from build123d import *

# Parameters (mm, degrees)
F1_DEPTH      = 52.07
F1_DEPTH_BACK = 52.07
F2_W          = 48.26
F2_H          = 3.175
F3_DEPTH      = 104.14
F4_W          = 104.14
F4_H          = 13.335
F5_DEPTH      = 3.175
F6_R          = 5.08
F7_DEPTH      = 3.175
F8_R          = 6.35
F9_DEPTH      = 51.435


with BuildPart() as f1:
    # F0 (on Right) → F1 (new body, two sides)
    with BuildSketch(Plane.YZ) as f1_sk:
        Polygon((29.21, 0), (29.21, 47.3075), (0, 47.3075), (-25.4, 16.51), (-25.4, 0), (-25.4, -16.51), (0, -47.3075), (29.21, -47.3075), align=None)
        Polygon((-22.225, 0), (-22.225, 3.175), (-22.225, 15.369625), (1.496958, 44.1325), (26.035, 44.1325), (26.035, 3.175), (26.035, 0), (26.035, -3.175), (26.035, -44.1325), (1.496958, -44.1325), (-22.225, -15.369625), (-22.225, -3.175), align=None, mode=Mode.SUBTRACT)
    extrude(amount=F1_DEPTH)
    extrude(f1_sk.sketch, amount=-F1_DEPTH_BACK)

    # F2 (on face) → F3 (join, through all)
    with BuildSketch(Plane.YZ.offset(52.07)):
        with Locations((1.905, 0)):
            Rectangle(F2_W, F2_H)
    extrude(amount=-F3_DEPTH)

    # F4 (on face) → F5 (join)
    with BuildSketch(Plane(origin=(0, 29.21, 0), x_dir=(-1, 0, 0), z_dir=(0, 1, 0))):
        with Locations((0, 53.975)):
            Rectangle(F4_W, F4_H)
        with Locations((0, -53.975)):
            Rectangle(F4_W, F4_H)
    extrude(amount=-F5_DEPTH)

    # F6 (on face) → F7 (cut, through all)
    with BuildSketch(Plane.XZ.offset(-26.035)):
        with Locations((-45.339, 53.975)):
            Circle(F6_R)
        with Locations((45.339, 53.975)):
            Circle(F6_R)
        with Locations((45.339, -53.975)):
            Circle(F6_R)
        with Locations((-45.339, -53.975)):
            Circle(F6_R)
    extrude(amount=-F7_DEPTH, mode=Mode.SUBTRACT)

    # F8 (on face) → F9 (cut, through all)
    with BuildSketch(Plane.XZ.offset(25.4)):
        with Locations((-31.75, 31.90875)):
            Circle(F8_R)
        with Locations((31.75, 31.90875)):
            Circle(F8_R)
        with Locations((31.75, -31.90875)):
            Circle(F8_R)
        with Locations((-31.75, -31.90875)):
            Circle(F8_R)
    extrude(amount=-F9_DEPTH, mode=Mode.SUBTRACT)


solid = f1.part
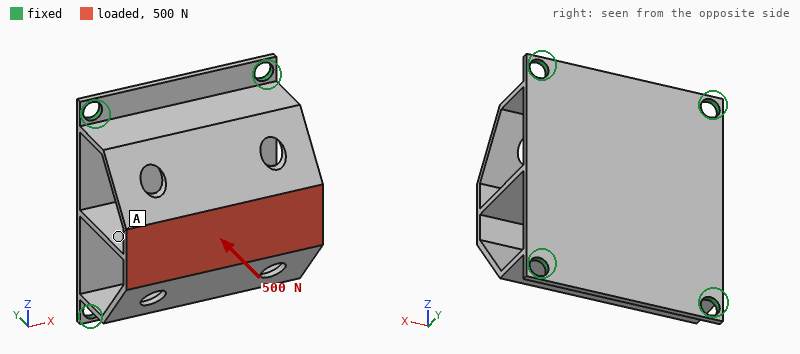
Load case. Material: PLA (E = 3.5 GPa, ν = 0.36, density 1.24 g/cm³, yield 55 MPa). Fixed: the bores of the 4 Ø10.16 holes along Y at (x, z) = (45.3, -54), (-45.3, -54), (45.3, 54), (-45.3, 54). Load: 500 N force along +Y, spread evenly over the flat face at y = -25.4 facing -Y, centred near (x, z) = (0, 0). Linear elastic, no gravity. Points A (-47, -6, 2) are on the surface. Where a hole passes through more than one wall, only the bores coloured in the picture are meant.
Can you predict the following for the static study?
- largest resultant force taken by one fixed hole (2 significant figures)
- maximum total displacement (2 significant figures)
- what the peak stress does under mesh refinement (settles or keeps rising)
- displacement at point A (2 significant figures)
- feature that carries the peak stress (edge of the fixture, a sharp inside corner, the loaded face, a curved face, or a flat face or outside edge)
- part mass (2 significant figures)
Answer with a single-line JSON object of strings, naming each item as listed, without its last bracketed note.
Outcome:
{"largest resultant force taken by one fixed hole": "140 N", "maximum total displacement": "0.51 mm", "what the peak stress does under mesh refinement": "keeps rising", "displacement at point A": "0.50 mm", "feature that carries the peak stress": "edge of the fixture", "part mass": "130 g"}
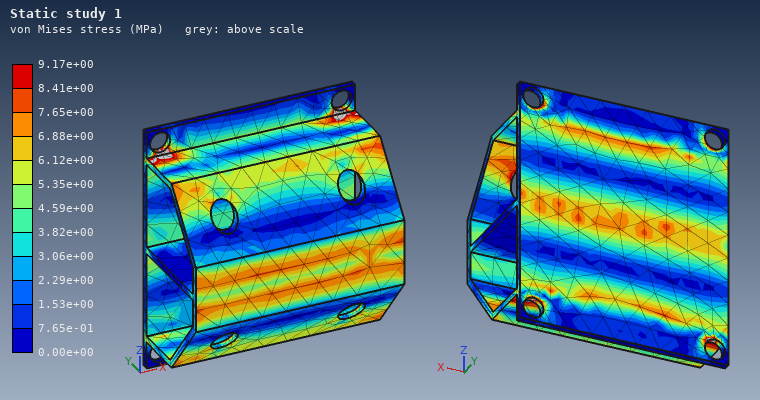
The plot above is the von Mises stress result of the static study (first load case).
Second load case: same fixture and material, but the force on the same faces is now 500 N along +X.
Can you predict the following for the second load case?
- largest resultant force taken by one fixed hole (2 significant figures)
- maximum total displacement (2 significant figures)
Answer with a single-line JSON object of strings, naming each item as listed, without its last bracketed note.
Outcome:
{"largest resultant force taken by one fixed hole": "200 N", "maximum total displacement": "0.38 mm"}
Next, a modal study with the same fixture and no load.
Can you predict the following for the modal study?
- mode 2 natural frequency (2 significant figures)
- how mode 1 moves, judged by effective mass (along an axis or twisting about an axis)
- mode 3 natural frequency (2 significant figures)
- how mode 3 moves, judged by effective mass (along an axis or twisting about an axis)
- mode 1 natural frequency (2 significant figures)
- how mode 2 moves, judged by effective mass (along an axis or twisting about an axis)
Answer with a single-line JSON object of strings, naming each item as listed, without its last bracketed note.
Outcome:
{"mode 2 natural frequency": "630 Hz", "how mode 1 moves, judged by effective mass": "along Z", "mode 3 natural frequency": "930 Hz", "how mode 3 moves, judged by effective mass": "along X", "mode 1 natural frequency": "450 Hz", "how mode 2 moves, judged by effective mass": "along Y"}
